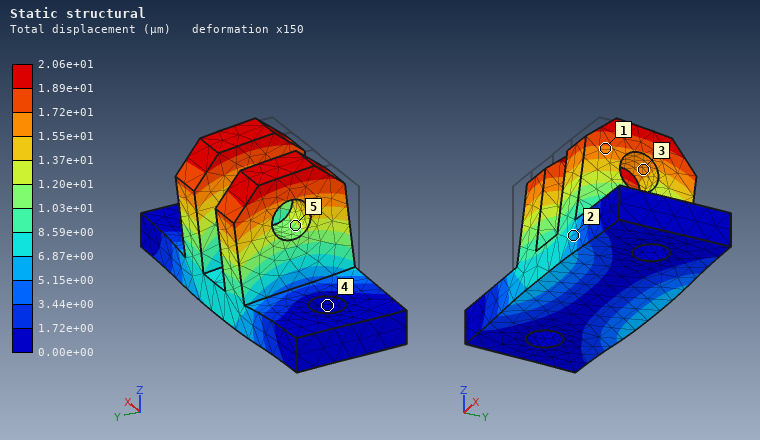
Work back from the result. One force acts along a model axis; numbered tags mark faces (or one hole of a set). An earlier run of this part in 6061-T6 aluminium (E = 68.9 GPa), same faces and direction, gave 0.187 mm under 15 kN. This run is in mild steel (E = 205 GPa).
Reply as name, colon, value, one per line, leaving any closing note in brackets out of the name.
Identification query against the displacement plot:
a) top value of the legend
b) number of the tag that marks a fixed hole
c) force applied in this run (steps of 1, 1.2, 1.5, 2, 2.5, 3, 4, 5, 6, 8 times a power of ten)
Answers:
top value of the legend: 2.06e+01 µm
number of the tag that marks a fixed hole: 4
force applied in this run: 5 kN
